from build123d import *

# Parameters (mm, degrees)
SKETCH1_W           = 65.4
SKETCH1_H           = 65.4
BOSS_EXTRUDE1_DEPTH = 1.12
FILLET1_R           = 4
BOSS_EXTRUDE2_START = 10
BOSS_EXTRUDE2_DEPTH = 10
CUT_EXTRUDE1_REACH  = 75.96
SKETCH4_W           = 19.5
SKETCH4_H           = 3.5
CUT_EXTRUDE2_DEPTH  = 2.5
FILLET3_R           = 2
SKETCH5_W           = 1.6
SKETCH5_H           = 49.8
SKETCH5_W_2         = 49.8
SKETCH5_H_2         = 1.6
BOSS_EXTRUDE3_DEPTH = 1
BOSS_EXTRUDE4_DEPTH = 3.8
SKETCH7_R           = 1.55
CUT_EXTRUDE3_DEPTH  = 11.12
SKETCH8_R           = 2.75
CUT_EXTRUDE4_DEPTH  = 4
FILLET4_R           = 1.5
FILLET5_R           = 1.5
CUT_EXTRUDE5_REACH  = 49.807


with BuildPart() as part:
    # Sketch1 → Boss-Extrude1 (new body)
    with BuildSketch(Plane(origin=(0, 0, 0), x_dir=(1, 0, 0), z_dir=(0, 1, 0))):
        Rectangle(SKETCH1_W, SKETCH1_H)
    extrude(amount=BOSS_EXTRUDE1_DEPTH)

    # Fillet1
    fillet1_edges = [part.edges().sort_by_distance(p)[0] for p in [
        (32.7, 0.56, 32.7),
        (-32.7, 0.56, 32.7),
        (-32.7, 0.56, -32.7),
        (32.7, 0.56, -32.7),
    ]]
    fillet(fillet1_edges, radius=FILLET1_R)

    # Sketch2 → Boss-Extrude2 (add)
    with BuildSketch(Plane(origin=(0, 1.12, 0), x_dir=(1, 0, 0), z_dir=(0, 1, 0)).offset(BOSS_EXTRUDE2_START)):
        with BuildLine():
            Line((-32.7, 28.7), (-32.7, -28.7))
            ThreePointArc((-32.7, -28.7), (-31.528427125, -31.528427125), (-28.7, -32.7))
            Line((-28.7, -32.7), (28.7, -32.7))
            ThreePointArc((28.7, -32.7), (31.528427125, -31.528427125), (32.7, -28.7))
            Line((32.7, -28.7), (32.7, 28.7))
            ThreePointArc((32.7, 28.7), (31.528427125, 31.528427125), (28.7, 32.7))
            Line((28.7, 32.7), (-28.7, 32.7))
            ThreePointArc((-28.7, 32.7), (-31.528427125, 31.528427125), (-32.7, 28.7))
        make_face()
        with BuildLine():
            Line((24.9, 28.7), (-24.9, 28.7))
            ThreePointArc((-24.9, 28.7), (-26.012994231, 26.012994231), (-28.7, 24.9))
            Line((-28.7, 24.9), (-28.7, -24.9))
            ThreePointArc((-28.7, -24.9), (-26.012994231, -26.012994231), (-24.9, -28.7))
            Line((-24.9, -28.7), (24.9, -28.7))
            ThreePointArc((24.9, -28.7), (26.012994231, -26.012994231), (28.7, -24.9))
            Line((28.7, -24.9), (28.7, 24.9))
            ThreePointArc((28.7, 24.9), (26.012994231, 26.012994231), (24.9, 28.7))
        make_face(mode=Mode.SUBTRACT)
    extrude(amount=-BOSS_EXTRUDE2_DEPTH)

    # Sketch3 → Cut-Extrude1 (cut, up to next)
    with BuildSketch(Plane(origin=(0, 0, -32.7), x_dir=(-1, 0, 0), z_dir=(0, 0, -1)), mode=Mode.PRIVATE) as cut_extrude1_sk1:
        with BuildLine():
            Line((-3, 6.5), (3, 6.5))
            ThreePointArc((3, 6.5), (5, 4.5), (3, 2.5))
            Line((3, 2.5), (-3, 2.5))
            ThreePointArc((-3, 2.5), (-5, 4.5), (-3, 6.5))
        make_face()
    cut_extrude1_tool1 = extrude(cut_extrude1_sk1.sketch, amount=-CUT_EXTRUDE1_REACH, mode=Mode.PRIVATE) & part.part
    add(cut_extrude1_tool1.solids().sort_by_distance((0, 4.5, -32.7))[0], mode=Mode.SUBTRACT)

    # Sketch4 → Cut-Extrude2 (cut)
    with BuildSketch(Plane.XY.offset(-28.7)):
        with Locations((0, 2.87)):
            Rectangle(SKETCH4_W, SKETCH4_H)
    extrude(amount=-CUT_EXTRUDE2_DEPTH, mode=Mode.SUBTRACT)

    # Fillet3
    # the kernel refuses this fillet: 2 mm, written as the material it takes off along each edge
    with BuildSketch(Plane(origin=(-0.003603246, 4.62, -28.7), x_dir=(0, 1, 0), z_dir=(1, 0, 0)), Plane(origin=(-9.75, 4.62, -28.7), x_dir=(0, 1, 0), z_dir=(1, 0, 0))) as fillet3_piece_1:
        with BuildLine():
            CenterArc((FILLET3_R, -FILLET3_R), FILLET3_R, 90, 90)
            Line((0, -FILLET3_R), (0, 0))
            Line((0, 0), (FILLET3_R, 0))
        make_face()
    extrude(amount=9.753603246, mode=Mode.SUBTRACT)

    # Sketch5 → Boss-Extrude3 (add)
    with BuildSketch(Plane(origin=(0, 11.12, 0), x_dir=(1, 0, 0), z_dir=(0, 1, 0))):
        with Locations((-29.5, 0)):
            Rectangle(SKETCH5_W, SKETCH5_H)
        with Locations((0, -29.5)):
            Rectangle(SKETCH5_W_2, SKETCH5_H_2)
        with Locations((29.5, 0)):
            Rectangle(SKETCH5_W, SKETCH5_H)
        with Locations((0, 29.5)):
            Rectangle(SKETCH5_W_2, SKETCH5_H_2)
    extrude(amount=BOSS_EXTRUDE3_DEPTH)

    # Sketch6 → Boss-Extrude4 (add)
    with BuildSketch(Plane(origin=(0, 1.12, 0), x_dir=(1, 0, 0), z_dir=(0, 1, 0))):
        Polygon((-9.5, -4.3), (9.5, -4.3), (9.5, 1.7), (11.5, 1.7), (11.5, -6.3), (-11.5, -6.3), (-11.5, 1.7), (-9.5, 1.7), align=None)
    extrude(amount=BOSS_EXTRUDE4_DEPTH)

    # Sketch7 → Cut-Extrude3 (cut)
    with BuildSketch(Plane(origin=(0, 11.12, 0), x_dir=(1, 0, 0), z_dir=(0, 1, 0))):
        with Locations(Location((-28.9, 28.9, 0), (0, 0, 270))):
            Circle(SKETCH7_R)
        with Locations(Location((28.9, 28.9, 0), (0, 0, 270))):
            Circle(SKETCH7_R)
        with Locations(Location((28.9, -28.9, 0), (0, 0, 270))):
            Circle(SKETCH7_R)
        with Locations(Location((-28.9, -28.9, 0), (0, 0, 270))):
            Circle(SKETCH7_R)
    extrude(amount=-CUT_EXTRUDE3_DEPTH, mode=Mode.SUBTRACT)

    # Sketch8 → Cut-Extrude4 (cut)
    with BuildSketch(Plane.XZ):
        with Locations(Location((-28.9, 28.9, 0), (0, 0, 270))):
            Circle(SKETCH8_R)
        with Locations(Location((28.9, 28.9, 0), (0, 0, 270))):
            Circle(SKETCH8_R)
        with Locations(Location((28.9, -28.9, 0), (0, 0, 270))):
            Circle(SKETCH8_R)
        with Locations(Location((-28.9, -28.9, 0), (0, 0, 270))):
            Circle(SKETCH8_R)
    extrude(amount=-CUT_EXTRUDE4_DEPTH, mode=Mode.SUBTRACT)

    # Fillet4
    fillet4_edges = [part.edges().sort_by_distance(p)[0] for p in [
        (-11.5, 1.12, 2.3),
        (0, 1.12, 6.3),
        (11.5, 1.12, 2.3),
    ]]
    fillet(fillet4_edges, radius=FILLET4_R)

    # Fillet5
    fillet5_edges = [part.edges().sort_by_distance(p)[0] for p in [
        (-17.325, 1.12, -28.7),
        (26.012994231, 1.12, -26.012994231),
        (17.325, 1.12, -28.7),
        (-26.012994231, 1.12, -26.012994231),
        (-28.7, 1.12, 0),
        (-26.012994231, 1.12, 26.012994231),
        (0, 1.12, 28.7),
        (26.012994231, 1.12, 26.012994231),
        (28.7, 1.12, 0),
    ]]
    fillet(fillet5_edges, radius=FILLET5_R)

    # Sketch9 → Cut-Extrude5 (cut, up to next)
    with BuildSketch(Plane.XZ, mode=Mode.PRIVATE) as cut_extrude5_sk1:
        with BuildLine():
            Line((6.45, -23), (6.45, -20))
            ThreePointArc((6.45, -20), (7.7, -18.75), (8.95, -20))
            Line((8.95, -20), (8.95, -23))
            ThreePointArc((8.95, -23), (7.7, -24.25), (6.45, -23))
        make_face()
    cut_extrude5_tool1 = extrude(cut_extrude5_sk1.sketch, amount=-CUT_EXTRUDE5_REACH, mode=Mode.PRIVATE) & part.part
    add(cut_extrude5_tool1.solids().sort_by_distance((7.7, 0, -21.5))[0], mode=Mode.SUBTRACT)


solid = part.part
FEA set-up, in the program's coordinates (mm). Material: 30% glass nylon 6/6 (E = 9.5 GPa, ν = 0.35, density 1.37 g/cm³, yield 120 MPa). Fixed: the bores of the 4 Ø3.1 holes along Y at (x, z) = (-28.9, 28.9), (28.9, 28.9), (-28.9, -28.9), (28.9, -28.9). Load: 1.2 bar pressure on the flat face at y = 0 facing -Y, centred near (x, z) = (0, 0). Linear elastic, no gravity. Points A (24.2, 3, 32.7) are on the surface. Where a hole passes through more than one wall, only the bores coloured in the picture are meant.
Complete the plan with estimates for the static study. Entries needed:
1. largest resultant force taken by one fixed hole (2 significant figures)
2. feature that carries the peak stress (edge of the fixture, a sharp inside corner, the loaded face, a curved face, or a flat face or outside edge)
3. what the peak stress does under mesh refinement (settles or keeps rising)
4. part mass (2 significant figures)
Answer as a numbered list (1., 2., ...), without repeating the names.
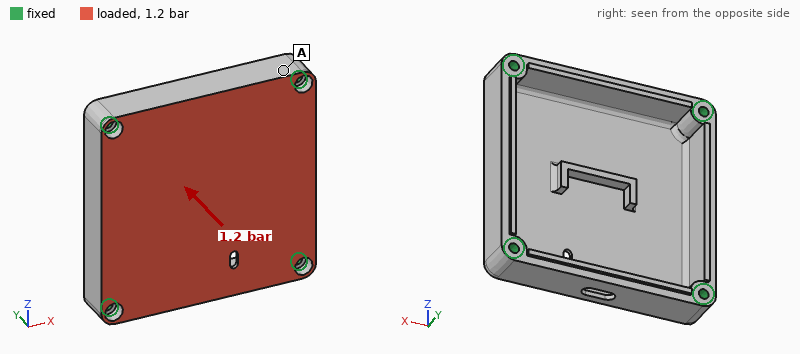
1. 160 N
2. a sharp inside corner
3. keeps rising
4. 20 g
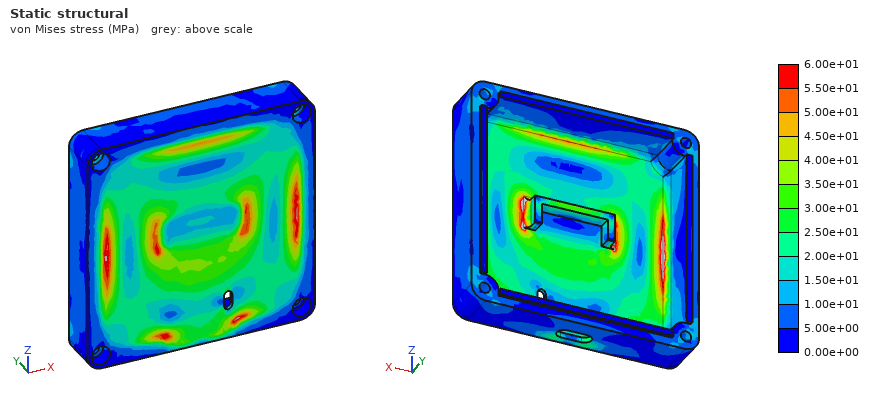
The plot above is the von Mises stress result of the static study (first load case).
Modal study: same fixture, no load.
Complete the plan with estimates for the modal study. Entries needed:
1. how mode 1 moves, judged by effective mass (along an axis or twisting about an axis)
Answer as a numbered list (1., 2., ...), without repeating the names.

1. along Y
